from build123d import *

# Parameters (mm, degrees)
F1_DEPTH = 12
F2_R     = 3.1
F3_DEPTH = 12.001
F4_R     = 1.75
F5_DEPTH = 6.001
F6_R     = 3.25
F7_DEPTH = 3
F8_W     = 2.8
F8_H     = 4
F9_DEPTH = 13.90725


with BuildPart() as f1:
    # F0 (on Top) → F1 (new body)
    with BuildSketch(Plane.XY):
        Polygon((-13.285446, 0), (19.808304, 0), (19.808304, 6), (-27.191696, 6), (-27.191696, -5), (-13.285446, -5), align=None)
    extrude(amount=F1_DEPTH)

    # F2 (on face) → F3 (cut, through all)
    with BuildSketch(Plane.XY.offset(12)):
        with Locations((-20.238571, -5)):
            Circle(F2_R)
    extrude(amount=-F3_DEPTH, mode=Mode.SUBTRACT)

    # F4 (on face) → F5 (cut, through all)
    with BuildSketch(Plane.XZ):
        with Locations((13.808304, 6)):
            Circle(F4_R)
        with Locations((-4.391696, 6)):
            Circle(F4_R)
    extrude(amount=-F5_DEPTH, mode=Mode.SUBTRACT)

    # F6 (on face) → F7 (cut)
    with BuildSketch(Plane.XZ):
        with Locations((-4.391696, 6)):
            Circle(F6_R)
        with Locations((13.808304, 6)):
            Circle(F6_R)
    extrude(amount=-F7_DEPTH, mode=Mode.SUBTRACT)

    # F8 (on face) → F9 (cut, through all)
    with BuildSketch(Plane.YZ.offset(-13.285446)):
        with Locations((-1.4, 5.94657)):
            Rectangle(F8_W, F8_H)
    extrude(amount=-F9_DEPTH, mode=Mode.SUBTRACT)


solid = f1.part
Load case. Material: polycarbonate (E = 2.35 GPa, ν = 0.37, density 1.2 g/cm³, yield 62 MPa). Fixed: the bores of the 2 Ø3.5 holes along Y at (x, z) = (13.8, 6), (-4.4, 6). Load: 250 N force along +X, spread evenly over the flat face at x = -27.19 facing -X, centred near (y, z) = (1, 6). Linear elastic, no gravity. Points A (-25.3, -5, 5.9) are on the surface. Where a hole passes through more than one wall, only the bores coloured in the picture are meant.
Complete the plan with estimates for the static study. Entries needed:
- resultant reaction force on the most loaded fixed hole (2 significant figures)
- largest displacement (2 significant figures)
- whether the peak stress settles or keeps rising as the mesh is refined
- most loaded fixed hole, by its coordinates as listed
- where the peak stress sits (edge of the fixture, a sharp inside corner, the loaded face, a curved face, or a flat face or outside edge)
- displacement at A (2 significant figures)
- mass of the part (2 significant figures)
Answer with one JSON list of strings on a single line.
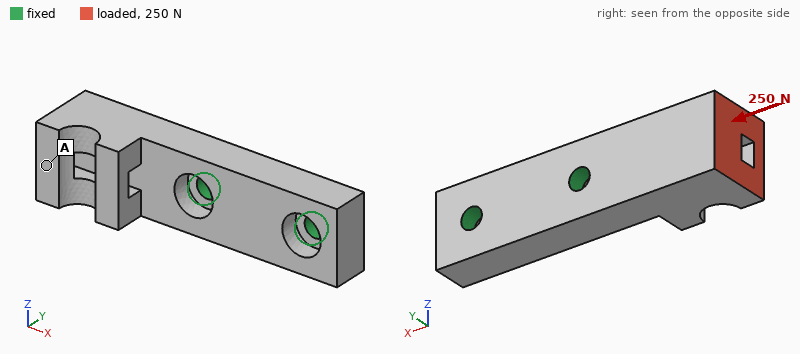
["160 N", "0.53 mm", "keeps rising", "(-4.4, 6)", "edge of the fixture", "0.48 mm", "4.4 g"]
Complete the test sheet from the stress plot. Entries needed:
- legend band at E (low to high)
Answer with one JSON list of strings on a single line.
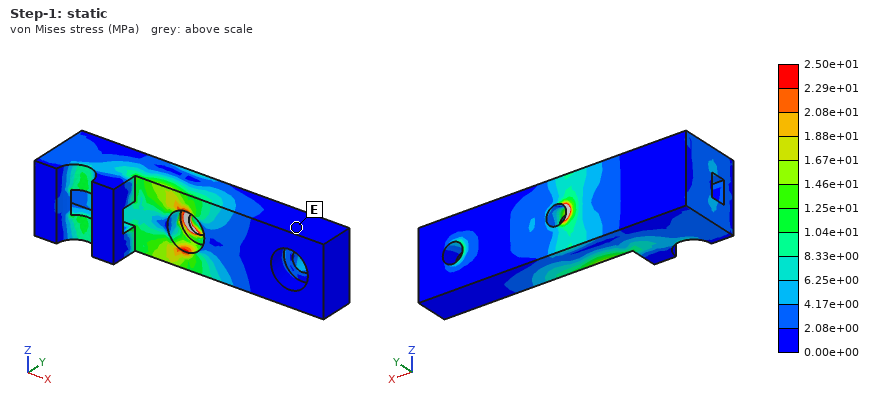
["0.00e+00 to 2.08e+00 MPa"]
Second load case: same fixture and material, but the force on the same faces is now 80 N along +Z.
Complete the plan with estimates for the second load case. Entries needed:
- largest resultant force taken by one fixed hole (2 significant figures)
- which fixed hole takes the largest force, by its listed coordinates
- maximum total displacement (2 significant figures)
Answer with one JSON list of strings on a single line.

["150 N", "(-4.4, 6)", "0.40 mm"]
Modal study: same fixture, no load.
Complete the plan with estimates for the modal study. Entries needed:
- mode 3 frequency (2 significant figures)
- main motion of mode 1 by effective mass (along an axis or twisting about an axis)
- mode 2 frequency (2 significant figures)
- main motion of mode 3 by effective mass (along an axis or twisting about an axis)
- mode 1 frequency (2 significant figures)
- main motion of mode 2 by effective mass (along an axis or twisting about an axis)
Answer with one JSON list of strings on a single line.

["4200 Hz", "along Y", "2500 Hz", "twisting about X", "1500 Hz", "along Z"]
